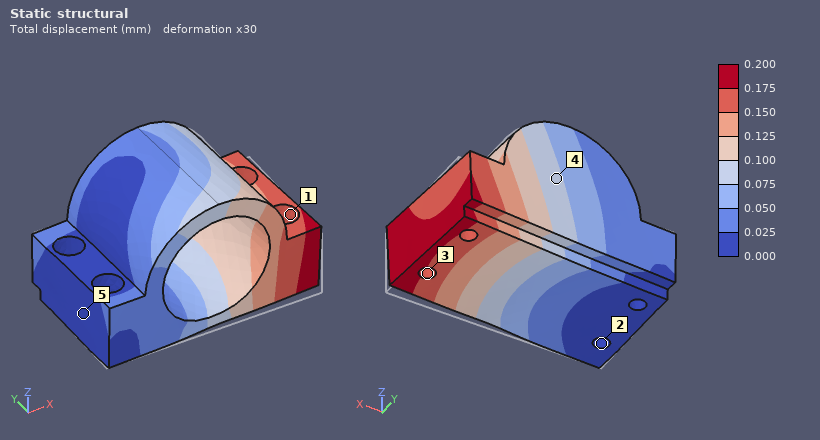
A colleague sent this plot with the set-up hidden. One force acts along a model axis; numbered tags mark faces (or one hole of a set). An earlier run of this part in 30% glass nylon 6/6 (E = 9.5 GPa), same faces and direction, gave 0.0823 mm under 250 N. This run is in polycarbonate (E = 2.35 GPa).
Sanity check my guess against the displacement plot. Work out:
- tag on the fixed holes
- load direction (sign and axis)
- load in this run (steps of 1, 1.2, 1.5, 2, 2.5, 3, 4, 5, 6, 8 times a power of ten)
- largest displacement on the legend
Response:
2
+Y
150 N
0.200 mm
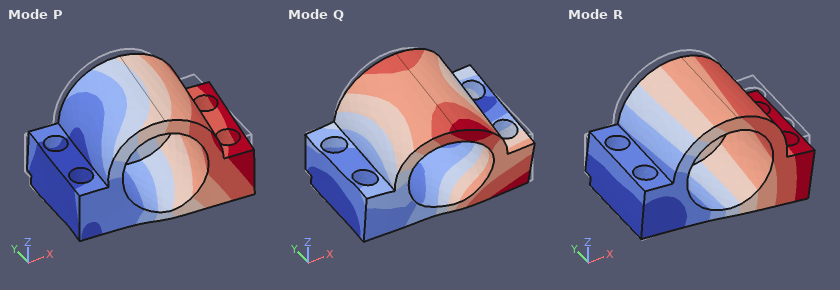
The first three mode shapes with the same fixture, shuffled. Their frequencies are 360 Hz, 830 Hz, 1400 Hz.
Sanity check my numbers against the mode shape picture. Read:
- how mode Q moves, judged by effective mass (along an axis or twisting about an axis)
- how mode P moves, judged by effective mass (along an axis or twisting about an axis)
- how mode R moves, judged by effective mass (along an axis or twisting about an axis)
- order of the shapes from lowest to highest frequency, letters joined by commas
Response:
twisting about X
along Y
along Z
R, P, Q
